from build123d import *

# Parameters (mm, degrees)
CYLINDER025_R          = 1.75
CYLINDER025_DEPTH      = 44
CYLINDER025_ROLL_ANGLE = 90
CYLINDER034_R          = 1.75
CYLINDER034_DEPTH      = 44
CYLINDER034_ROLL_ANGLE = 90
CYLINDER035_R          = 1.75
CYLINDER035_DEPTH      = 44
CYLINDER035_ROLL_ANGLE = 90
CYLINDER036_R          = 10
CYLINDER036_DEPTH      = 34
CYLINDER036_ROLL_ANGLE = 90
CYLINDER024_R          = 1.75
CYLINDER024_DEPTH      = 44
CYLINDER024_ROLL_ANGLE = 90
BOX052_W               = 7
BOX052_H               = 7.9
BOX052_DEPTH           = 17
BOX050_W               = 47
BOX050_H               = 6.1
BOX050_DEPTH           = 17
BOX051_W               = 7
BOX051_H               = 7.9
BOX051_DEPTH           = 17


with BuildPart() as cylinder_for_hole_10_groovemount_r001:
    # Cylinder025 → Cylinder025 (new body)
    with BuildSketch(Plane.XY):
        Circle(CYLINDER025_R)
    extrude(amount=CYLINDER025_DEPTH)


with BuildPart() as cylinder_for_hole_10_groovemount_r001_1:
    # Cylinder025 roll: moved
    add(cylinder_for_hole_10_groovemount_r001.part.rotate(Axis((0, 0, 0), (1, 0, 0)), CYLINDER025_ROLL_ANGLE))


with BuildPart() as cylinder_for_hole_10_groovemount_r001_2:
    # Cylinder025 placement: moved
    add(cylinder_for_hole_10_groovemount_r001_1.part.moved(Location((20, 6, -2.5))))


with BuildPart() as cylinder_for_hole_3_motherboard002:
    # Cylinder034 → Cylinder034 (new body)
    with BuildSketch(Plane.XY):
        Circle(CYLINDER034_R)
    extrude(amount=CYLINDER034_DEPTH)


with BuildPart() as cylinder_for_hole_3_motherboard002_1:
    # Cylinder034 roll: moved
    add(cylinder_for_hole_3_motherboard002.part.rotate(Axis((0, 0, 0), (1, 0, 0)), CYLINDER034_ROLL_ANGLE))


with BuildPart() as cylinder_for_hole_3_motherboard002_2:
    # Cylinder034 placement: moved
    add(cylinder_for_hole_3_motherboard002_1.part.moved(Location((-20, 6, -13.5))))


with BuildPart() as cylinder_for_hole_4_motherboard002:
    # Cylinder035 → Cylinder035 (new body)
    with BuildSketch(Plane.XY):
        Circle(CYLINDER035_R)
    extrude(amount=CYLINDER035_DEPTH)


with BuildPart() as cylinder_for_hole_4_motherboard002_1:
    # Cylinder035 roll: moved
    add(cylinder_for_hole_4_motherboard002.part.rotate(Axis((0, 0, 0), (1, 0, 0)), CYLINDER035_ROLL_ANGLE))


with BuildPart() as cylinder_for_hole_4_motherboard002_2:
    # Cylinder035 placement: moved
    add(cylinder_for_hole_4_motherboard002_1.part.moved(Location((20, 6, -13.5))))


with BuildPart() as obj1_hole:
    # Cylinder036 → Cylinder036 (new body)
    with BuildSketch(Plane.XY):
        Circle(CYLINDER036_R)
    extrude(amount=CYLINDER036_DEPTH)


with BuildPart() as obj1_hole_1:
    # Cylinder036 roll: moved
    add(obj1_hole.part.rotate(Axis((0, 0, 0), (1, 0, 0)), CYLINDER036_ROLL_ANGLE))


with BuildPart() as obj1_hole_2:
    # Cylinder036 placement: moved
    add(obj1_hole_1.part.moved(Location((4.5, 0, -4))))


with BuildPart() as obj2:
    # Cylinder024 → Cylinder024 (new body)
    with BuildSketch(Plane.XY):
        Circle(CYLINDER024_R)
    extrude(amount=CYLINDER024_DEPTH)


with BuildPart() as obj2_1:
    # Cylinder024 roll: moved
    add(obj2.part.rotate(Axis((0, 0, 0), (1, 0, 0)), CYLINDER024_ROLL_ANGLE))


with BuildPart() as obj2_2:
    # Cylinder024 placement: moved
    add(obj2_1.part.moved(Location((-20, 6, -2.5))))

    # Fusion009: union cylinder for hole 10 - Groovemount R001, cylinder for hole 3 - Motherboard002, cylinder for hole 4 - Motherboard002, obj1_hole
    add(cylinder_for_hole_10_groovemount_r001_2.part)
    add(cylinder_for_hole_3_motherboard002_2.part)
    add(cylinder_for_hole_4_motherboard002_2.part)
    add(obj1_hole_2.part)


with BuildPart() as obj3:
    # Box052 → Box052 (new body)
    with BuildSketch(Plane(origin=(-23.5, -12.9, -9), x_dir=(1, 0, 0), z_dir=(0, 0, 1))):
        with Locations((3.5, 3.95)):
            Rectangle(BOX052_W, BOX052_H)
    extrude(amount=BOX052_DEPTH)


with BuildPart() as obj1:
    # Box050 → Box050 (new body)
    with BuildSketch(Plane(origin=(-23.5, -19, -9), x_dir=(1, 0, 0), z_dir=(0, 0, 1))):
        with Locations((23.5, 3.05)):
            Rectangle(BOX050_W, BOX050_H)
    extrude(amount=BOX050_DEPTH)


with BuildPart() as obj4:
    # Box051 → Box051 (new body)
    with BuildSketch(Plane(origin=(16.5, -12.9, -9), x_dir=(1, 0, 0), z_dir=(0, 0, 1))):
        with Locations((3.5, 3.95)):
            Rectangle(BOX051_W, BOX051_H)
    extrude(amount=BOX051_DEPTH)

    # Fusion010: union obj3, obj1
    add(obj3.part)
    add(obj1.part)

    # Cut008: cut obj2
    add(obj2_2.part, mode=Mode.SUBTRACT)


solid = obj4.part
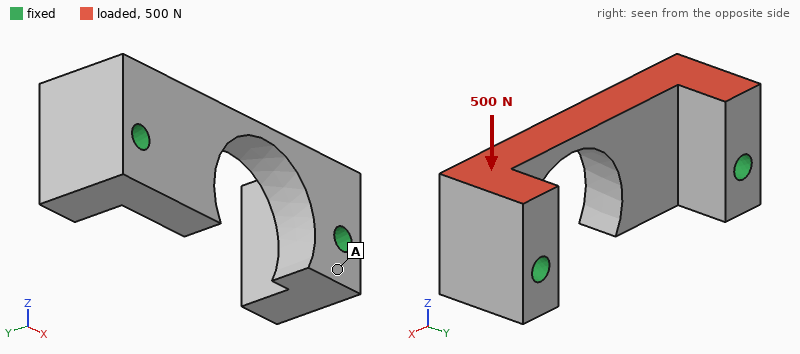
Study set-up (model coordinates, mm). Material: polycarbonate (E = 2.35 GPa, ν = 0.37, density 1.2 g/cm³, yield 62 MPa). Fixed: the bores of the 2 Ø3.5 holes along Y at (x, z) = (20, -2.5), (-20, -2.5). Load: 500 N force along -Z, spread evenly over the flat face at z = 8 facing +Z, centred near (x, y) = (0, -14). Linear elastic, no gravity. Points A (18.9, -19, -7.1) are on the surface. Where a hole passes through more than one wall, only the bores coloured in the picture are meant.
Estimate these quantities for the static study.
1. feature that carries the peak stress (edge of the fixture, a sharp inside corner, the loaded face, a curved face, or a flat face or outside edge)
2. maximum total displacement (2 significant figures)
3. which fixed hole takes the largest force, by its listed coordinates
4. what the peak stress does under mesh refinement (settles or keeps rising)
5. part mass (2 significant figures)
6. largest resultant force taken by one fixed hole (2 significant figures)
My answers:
edge of the fixture
0.11 mm
(-20, -2.5)
keeps rising
5.9 g
290 N
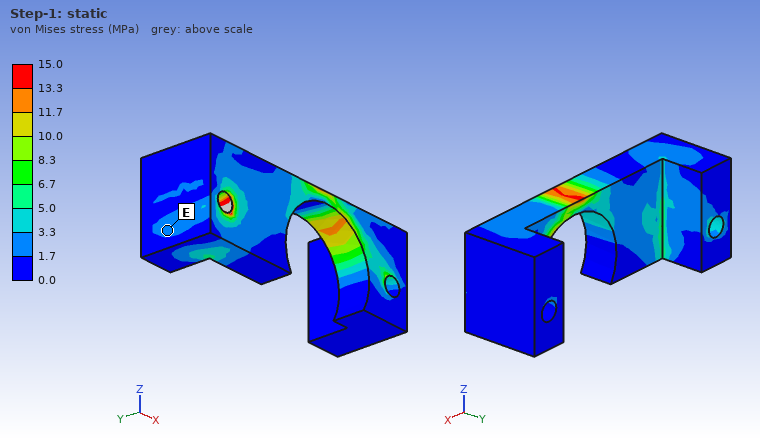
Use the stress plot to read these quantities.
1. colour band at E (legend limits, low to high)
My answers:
1.7 to 3.3 MPa
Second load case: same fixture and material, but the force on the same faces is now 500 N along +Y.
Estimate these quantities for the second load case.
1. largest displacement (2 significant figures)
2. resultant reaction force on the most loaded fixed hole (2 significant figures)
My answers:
0.31 mm
260 N
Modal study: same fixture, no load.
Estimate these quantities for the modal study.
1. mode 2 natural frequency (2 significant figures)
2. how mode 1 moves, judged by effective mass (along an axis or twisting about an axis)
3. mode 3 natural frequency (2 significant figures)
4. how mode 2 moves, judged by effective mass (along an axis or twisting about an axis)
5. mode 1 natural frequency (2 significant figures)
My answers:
6000 Hz
along Y
9000 Hz
along Z
5700 Hz
